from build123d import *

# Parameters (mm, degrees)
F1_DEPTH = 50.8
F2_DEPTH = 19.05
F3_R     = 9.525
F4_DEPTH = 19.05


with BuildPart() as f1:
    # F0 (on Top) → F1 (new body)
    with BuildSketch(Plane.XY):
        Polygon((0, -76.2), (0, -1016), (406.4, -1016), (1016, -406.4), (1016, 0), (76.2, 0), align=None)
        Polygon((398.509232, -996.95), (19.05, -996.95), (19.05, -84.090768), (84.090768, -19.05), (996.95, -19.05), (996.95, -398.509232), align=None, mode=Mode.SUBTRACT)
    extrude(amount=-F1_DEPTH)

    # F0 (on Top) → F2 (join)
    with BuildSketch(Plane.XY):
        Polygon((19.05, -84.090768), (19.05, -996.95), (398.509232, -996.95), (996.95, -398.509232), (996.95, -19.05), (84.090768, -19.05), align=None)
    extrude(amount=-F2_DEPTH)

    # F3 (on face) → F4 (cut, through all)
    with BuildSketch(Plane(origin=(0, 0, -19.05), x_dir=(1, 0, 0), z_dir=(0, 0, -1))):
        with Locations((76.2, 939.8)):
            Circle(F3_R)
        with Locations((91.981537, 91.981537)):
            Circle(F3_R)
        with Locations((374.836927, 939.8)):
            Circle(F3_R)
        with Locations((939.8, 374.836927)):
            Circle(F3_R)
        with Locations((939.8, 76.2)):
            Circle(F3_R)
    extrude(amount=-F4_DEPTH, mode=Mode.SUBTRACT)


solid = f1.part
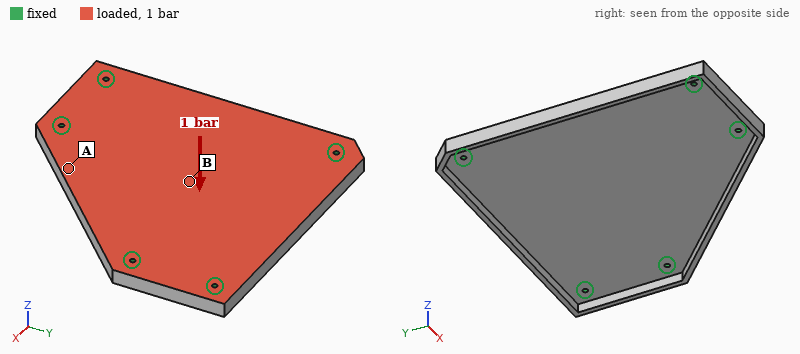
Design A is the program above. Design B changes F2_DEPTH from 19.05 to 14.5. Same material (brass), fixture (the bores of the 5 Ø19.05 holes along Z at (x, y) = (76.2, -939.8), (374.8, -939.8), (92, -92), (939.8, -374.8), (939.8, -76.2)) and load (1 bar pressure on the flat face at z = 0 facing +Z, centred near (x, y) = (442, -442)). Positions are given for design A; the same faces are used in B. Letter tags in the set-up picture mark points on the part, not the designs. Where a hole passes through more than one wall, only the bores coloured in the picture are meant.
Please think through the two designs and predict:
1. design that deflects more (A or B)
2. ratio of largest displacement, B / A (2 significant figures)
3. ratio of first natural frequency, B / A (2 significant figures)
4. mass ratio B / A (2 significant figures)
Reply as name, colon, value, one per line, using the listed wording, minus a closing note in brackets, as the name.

design that deflects more: B
ratio of largest displacement, B / A: 2.0
ratio of first natural frequency, B / A: 0.83
mass ratio B / A: 0.81
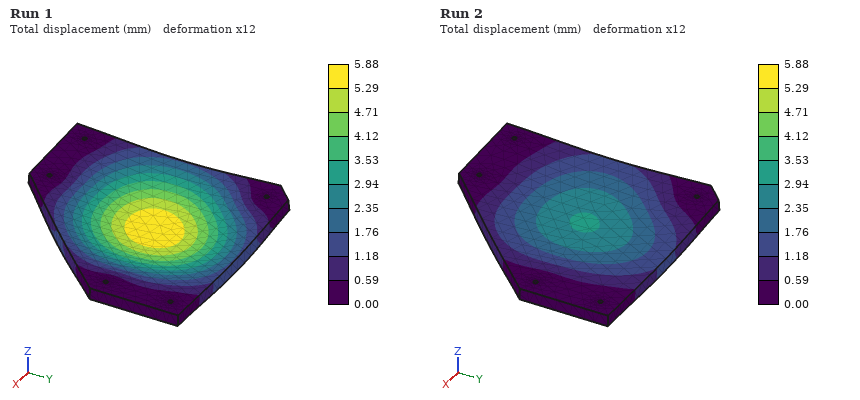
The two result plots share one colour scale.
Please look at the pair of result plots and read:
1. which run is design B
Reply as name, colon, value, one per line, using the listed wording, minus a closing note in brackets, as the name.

which run is design B: Run 1
